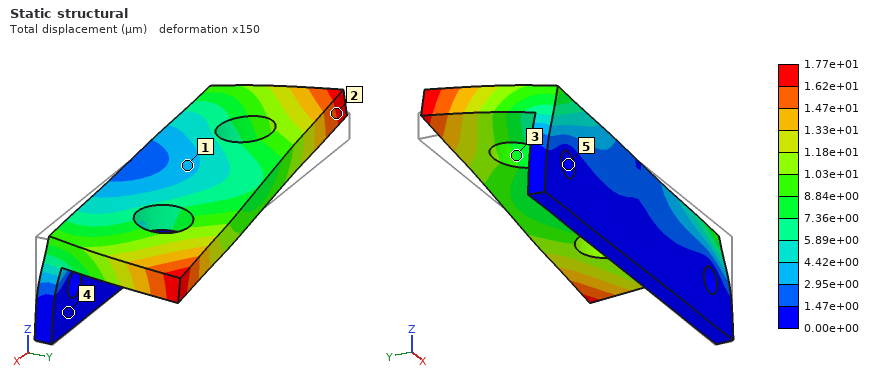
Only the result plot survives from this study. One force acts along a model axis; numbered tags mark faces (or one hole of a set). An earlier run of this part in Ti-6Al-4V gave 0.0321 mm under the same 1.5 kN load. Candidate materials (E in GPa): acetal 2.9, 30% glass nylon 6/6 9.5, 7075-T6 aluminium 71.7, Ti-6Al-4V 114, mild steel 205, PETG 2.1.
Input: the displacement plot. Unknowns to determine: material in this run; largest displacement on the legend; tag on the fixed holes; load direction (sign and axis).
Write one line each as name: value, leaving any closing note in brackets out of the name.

material in this run: mild steel
largest displacement on the legend: 1.77e+01 µm
tag on the fixed holes: 5
load direction: -X
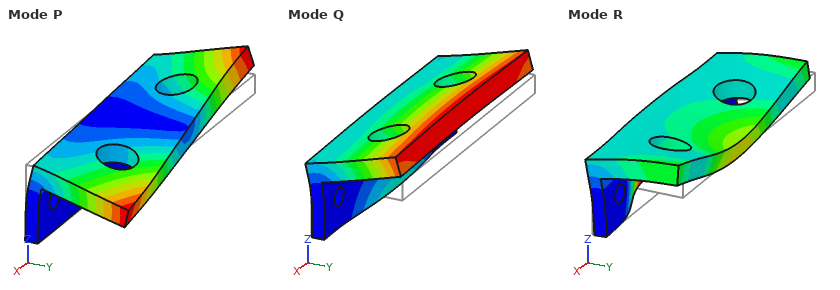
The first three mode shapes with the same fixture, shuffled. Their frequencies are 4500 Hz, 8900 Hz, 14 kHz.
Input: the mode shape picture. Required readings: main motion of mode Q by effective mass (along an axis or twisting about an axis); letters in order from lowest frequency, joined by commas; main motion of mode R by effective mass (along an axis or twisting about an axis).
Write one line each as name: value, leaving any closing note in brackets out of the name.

main motion of mode Q by effective mass: along Z
letters in order from lowest frequency, joined by commas: Q, P, R
main motion of mode R by effective mass: along Y
